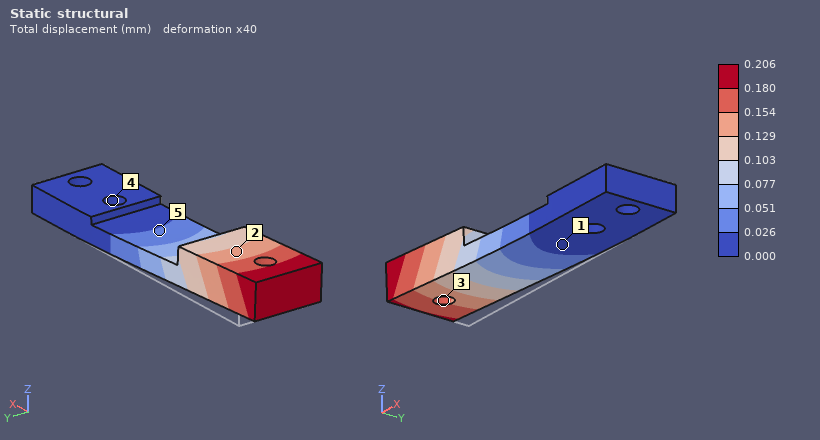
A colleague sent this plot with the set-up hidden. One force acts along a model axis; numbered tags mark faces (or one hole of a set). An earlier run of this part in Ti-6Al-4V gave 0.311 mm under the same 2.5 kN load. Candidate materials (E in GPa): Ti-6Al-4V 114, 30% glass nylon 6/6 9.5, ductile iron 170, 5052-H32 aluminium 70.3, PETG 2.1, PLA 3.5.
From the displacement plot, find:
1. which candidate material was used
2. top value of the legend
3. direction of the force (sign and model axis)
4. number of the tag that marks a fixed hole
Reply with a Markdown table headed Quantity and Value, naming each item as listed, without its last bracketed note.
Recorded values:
| Quantity | Value |
|---|---|
| which candidate material was used | ductile iron |
| top value of the legend | 0.206 mm |
| direction of the force | -Y |
| number of the tag that marks a fixed hole | 4 |
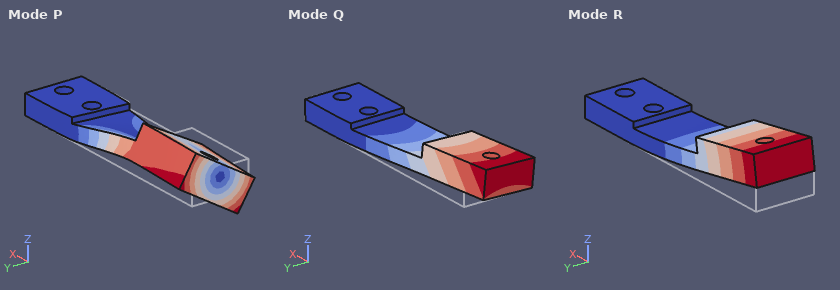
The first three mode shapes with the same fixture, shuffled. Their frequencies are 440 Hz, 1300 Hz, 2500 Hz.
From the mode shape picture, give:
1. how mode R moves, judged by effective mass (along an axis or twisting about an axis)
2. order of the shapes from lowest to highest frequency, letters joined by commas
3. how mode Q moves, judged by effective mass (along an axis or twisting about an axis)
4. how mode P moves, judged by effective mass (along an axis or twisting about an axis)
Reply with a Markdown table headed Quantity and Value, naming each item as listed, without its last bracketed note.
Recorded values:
| Quantity | Value |
|---|---|
| how mode R moves, judged by effective mass | along Z |
| order of the shapes from lowest to highest frequency, letters joined by commas | R, Q, P |
| how mode Q moves, judged by effective mass | along Y |
| how mode P moves, judged by effective mass | twisting about X |
